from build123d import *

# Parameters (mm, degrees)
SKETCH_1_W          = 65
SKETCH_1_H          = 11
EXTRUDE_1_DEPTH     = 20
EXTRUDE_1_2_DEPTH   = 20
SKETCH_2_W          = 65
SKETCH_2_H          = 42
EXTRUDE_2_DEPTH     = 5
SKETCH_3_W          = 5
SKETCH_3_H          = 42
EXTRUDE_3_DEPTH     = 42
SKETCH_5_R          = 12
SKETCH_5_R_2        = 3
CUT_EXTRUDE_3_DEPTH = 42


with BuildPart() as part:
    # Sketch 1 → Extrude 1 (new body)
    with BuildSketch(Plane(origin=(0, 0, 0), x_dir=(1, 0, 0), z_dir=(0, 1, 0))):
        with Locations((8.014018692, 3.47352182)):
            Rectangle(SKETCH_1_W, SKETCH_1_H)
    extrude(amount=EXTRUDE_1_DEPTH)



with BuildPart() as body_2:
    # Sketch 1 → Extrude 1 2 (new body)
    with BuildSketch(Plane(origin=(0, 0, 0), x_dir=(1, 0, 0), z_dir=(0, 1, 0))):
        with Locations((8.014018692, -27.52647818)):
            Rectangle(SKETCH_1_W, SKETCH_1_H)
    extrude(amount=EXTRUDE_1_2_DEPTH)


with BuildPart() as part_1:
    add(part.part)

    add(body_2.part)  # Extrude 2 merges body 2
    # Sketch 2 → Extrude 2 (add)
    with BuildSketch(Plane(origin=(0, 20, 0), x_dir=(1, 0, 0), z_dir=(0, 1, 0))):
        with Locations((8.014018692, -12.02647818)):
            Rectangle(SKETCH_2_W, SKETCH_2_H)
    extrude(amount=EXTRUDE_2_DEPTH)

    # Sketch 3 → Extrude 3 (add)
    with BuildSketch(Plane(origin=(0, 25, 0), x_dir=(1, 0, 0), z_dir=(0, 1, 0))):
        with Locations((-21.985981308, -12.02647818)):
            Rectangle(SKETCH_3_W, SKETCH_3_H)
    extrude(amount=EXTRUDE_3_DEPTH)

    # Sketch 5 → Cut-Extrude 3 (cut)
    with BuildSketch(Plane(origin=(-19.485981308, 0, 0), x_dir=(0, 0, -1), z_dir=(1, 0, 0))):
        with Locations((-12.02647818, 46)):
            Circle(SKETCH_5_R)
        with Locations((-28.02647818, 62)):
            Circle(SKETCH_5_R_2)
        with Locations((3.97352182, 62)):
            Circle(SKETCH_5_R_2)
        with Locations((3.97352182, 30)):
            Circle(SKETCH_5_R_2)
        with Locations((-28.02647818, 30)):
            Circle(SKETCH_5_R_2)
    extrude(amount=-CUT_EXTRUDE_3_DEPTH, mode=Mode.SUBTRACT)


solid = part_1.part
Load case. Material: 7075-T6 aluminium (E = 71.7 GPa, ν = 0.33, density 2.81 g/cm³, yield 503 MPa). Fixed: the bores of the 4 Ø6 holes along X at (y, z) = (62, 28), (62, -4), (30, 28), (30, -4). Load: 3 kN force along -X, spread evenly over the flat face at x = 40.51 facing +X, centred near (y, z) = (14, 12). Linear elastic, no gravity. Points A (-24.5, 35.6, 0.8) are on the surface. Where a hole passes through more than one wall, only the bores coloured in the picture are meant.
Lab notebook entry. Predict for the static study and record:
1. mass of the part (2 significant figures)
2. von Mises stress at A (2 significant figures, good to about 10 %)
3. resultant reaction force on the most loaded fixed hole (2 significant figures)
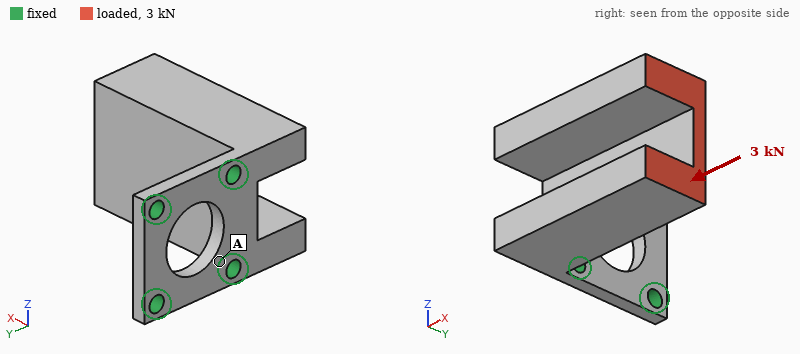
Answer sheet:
140 g
36 MPa
1.5 kN
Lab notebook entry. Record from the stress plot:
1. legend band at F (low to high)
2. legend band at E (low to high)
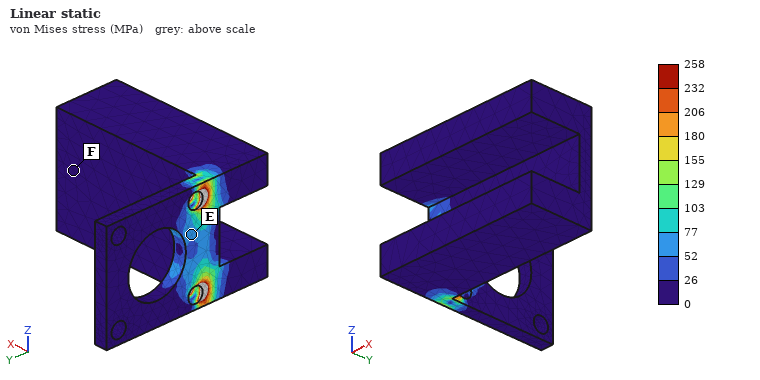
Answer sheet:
0 to 26 MPa
52 to 77 MPa
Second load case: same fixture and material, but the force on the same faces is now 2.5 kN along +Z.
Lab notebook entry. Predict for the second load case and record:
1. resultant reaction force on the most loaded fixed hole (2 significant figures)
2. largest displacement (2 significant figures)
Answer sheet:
5.0 kN
0.23 mm
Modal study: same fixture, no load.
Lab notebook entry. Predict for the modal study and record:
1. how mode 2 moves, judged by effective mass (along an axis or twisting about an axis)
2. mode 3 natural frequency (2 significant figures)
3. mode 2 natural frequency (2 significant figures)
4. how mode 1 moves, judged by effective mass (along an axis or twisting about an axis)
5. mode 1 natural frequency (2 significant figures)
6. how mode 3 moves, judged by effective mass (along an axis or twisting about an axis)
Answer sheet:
along Z
2900 Hz
2700 Hz
along Y
770 Hz
along Z
